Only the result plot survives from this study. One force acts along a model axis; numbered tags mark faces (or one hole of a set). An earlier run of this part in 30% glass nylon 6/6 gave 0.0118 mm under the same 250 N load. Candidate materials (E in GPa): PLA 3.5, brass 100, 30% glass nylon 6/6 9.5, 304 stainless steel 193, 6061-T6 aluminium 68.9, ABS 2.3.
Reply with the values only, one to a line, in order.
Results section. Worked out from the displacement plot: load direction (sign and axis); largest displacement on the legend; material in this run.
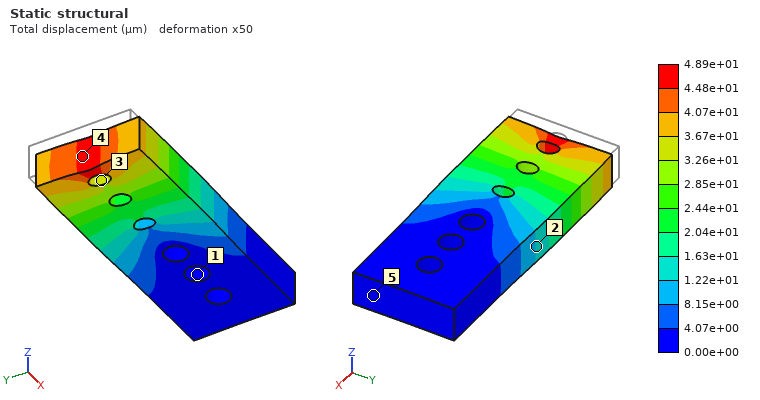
+X
4.89e+01 µm
ABS
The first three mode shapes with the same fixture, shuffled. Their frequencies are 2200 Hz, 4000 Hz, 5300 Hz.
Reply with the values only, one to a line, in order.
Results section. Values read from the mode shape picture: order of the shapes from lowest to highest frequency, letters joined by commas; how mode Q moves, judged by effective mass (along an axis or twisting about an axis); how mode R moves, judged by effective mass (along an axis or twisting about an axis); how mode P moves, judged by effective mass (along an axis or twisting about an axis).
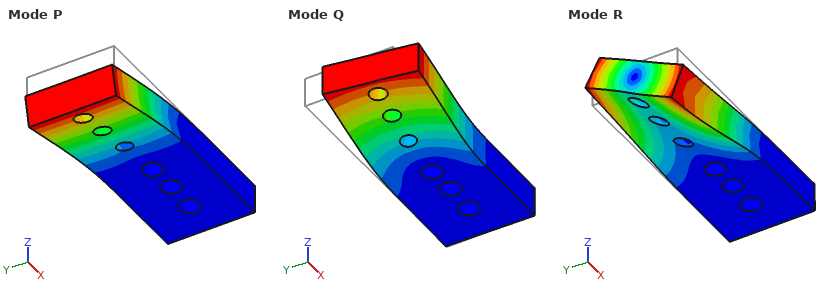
P, Q, R
along Y
twisting about X
along Z
